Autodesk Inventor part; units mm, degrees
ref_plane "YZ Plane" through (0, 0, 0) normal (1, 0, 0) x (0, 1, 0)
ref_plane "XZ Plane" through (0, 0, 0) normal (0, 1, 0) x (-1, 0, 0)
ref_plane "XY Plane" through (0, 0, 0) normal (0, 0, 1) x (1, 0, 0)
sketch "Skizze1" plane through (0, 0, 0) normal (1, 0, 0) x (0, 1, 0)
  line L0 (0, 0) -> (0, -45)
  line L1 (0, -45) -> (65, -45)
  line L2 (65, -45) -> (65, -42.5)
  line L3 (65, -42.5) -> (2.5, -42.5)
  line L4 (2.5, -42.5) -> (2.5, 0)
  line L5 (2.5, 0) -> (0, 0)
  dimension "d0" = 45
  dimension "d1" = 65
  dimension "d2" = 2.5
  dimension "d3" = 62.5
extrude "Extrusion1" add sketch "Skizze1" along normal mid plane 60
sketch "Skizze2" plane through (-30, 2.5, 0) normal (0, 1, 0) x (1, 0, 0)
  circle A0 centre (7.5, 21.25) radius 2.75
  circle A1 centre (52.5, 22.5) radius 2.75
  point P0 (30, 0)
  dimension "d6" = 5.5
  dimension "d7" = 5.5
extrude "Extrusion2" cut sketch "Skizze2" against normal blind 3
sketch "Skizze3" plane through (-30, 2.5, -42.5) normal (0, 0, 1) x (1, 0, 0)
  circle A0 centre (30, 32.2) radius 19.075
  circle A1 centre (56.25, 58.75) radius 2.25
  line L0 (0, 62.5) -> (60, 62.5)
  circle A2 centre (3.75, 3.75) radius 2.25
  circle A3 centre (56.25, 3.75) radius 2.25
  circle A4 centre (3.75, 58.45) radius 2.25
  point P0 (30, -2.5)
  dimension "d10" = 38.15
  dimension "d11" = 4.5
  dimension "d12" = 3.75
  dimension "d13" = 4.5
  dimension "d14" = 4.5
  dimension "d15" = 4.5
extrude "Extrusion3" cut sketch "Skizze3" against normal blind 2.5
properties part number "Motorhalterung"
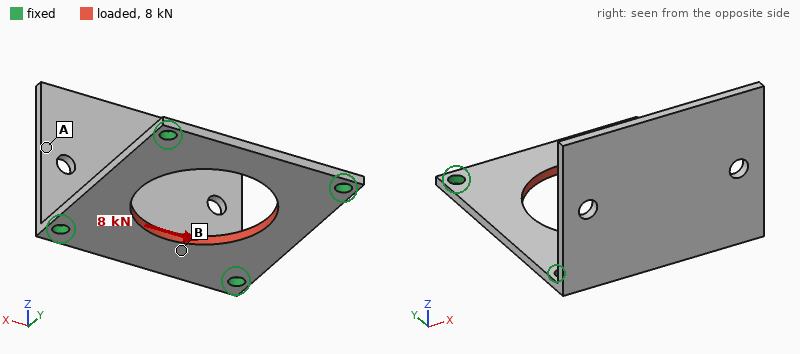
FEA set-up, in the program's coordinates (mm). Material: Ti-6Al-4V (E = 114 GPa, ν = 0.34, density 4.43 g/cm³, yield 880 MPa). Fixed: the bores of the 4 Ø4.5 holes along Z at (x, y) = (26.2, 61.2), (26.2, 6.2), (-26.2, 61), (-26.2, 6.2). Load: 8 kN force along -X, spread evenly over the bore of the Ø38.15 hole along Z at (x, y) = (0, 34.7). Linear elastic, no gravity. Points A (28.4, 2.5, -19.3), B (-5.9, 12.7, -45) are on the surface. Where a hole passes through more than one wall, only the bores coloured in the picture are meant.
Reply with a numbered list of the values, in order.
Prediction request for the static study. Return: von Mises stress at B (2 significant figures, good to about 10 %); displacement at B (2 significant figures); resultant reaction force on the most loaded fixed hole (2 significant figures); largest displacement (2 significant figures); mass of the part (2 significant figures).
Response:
1. 61 MPa
2. 9.7 µm
3. 2.2 kN
4. 31 µm
5. 58 g
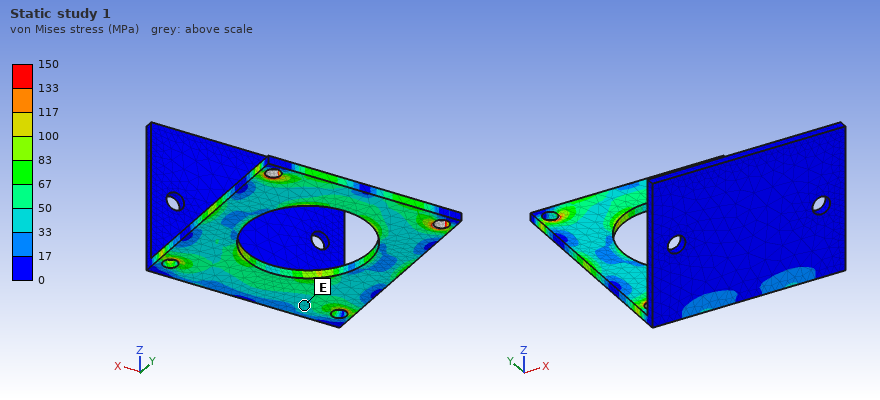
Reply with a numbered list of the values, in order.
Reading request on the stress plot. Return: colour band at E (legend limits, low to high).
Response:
1. 33 to 50 MPa
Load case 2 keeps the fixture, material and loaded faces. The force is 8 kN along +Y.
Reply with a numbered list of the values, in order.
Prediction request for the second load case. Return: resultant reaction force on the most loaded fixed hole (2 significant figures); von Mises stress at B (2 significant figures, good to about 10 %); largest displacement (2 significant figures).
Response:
1. 2.1 kN
2. 28 MPa
3. 34 µm
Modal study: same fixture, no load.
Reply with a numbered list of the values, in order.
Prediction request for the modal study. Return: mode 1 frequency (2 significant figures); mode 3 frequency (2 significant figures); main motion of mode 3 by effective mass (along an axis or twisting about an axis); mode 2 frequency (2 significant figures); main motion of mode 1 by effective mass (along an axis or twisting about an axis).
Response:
1. 870 Hz
2. 4600 Hz
3. along Z
4. 2000 Hz
5. along Y
